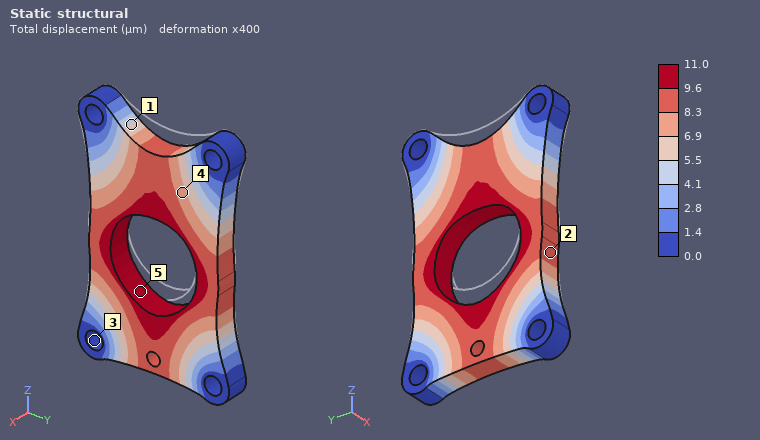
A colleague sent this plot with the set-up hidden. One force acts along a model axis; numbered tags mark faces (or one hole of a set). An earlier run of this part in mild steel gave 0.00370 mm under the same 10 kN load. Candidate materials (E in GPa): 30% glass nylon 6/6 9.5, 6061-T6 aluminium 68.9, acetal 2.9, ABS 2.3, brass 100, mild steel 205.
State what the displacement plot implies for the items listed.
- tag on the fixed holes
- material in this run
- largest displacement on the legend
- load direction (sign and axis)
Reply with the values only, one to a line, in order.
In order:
3
6061-T6 aluminium
11.0 µm
-Z
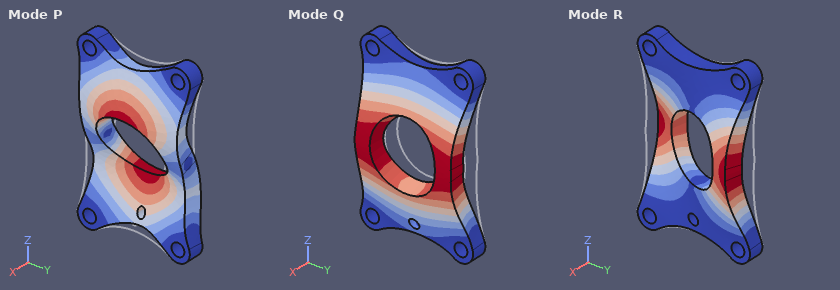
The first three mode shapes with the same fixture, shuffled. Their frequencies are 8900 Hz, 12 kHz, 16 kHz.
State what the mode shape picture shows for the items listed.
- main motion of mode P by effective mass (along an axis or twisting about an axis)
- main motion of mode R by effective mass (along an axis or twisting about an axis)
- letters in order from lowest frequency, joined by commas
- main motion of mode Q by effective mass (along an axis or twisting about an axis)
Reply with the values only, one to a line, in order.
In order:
twisting about Y
twisting about Z
Q, R, P
along X
